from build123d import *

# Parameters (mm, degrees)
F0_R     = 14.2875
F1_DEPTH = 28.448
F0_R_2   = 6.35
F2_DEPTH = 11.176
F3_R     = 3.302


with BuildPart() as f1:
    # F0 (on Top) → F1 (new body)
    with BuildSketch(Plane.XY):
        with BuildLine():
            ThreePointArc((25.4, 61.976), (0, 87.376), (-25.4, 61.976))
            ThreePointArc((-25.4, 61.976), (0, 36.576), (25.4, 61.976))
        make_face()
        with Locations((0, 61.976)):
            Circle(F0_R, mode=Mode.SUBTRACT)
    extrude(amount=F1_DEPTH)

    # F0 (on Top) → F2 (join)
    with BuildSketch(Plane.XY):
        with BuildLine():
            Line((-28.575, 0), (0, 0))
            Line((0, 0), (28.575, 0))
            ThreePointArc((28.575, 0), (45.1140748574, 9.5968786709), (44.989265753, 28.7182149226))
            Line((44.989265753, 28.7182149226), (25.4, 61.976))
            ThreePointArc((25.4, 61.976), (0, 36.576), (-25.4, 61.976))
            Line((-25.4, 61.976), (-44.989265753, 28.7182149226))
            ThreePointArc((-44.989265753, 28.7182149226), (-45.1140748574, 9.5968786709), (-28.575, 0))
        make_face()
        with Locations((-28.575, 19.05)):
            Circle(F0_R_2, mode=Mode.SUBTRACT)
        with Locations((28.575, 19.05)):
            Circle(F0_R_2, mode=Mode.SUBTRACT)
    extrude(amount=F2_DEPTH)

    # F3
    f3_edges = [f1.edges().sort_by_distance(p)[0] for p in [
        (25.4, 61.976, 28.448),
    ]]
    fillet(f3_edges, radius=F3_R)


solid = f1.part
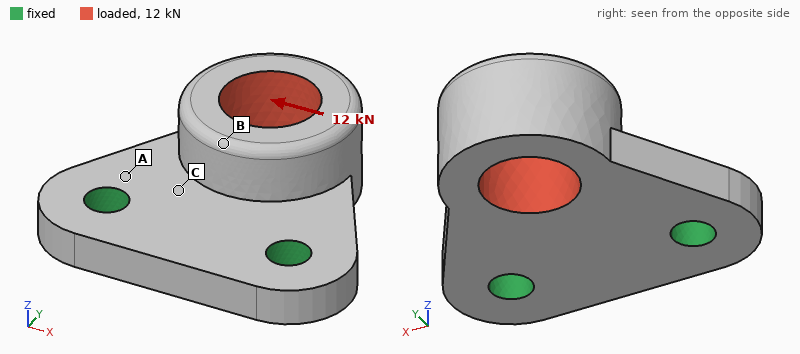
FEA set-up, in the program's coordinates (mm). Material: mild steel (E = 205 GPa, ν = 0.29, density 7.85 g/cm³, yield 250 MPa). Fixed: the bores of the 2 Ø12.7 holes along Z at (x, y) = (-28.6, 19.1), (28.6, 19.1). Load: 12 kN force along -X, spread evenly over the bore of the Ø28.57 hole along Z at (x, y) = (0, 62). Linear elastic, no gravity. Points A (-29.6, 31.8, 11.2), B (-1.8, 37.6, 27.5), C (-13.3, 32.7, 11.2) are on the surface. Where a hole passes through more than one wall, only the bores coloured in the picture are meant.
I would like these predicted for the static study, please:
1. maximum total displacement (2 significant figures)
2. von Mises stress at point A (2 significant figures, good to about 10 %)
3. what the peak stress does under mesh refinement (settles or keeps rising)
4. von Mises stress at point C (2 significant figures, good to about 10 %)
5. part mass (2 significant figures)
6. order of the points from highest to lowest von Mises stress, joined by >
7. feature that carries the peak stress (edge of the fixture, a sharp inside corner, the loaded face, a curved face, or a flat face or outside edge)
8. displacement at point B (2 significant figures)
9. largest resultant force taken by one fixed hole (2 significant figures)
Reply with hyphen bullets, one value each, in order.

- 26 µm
- 22 MPa
- keeps rising
- 43 MPa
- 630 g
- C > A > B
- edge of the fixture
- 13 µm
- 10.0 kN
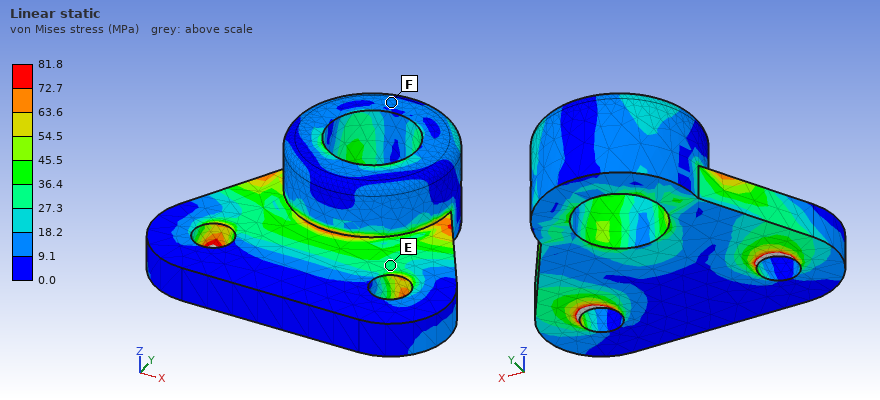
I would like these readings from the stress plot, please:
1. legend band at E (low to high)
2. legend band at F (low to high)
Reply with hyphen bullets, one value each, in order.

- 27.3 to 36.4 MPa
- 9.1 to 18.2 MPa
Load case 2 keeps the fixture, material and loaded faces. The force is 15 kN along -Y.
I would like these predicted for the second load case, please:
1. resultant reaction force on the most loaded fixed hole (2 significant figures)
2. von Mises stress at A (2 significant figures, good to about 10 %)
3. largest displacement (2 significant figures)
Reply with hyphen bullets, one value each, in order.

- 7.8 kN
- 99 MPa
- 0.11 mm
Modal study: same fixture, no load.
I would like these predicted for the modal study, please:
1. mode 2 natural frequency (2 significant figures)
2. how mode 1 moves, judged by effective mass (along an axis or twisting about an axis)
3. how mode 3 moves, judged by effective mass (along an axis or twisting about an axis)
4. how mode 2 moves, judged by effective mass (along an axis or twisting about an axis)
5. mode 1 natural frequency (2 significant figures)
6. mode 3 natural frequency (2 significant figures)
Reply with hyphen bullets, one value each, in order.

- 6500 Hz
- along Z
- along X
- along X
- 2100 Hz
- 8100 Hz
